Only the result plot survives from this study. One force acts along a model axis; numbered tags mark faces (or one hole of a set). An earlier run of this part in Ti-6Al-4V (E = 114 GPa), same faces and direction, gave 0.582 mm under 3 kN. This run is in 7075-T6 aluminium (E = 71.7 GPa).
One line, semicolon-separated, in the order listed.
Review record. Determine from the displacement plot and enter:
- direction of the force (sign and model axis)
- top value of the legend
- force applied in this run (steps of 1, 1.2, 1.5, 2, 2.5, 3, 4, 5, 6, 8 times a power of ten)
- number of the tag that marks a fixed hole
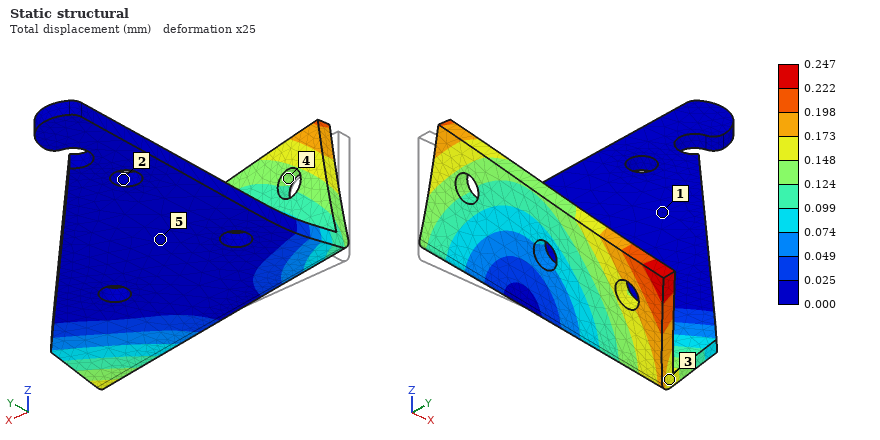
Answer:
+X; 0.247 mm; 800 N; 2
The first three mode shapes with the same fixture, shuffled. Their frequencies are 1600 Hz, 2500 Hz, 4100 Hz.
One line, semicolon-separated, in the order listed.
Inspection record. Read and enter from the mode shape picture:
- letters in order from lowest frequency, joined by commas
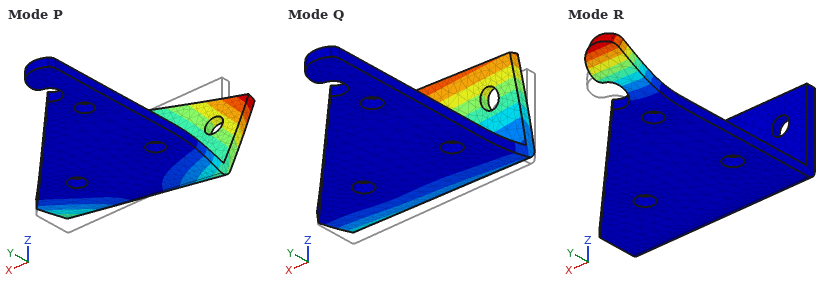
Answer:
Q, P, R
